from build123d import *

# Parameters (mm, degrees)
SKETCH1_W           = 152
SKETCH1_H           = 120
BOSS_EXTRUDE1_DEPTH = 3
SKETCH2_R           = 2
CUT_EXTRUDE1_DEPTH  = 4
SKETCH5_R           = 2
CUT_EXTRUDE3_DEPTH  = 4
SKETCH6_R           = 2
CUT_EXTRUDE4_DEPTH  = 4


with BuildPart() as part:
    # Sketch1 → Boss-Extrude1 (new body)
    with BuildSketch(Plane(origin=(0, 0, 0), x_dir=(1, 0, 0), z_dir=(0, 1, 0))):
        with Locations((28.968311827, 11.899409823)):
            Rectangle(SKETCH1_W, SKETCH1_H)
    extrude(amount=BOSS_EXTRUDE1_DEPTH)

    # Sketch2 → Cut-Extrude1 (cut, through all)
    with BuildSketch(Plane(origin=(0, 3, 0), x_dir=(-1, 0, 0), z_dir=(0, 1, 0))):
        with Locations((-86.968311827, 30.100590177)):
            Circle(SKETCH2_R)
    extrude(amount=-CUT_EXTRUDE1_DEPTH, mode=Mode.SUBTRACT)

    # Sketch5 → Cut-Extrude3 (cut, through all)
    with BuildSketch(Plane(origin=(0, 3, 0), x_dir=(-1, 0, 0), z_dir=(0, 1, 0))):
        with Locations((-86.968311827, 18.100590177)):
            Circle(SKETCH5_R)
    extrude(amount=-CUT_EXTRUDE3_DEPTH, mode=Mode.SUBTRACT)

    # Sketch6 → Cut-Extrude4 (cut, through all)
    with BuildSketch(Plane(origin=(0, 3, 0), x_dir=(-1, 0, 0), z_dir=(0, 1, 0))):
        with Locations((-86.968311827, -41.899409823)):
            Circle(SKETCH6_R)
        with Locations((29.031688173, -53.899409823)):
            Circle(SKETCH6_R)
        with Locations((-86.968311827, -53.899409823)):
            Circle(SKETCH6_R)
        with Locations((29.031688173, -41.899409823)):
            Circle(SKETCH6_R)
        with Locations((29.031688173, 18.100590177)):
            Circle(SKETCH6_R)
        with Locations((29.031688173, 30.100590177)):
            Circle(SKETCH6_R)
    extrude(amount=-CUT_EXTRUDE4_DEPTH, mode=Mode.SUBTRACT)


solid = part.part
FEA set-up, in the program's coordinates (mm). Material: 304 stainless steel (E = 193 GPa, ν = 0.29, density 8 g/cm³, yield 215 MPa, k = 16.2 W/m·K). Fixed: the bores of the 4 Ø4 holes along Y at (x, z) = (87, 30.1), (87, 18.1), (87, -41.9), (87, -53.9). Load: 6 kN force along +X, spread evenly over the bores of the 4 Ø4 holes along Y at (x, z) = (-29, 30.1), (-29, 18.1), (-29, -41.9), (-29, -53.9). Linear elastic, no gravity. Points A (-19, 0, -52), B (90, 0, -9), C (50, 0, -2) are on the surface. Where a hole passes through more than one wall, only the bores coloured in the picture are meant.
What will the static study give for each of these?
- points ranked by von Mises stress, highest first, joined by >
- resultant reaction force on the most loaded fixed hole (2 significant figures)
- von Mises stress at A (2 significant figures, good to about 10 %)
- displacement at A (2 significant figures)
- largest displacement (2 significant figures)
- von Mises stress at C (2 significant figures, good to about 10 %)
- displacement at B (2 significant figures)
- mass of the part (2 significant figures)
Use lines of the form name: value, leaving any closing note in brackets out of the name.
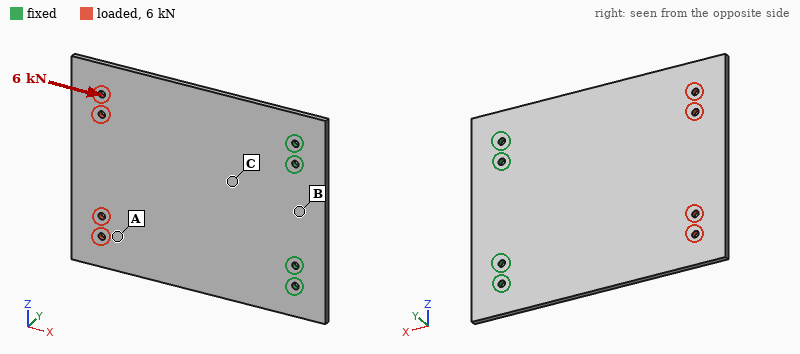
points ranked by von Mises stress, highest first, joined by >: A > C > B
resultant reaction force on the most loaded fixed hole: 1.6 kN
von Mises stress at A: 29 MPa
displacement at A: 12 µm
largest displacement: 14 µm
von Mises stress at C: 14 MPa
displacement at B: 3.1 µm
mass of the part: 440 g
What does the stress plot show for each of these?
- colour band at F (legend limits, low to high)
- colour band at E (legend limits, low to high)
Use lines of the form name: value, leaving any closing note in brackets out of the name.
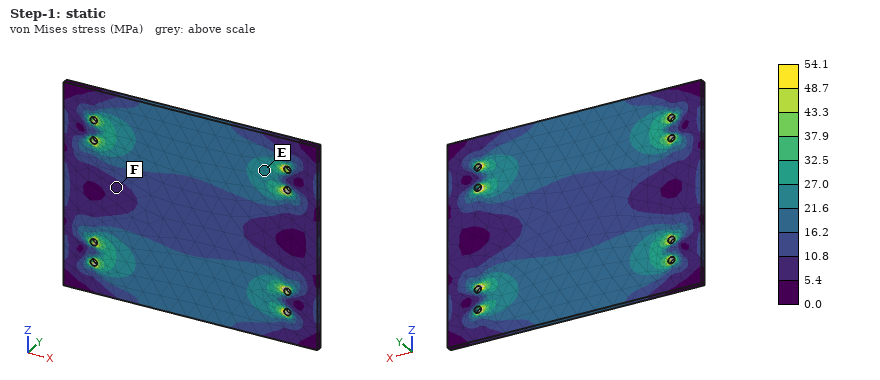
colour band at F: 5.4 to 10.8 MPa
colour band at E: 21.6 to 27.0 MPa
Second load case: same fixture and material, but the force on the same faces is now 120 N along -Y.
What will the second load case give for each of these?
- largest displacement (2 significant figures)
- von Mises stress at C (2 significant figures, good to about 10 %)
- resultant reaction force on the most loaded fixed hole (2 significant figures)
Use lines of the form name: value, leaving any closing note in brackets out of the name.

largest displacement: 1.5 mm
von Mises stress at C: 48 MPa
resultant reaction force on the most loaded fixed hole: 77 N
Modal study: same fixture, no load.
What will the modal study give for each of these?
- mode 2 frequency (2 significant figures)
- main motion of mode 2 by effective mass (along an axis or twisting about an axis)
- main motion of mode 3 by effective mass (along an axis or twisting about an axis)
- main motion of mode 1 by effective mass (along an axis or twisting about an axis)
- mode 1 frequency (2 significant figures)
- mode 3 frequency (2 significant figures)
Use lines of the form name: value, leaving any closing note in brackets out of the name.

mode 2 frequency: 360 Hz
main motion of mode 2 by effective mass: twisting about X
main motion of mode 3 by effective mass: along Y
main motion of mode 1 by effective mass: along Y
mode 1 frequency: 130 Hz
mode 3 frequency: 810 Hz
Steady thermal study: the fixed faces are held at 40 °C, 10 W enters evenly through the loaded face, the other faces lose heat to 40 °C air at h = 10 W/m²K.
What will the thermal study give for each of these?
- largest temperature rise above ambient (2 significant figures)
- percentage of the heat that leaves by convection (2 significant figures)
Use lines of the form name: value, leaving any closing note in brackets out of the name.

largest temperature rise above ambient: 77 K
percentage of the heat that leaves by convection: 89 %
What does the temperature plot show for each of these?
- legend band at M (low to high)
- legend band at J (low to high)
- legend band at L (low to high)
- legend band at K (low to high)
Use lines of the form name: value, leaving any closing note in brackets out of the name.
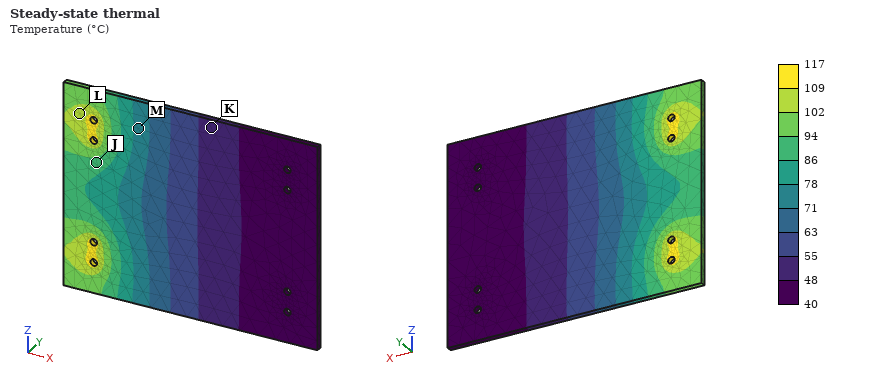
legend band at M: 71 to 78 °C
legend band at J: 86 to 94 °C
legend band at L: 102 to 109 °C
legend band at K: 48 to 55 °C
